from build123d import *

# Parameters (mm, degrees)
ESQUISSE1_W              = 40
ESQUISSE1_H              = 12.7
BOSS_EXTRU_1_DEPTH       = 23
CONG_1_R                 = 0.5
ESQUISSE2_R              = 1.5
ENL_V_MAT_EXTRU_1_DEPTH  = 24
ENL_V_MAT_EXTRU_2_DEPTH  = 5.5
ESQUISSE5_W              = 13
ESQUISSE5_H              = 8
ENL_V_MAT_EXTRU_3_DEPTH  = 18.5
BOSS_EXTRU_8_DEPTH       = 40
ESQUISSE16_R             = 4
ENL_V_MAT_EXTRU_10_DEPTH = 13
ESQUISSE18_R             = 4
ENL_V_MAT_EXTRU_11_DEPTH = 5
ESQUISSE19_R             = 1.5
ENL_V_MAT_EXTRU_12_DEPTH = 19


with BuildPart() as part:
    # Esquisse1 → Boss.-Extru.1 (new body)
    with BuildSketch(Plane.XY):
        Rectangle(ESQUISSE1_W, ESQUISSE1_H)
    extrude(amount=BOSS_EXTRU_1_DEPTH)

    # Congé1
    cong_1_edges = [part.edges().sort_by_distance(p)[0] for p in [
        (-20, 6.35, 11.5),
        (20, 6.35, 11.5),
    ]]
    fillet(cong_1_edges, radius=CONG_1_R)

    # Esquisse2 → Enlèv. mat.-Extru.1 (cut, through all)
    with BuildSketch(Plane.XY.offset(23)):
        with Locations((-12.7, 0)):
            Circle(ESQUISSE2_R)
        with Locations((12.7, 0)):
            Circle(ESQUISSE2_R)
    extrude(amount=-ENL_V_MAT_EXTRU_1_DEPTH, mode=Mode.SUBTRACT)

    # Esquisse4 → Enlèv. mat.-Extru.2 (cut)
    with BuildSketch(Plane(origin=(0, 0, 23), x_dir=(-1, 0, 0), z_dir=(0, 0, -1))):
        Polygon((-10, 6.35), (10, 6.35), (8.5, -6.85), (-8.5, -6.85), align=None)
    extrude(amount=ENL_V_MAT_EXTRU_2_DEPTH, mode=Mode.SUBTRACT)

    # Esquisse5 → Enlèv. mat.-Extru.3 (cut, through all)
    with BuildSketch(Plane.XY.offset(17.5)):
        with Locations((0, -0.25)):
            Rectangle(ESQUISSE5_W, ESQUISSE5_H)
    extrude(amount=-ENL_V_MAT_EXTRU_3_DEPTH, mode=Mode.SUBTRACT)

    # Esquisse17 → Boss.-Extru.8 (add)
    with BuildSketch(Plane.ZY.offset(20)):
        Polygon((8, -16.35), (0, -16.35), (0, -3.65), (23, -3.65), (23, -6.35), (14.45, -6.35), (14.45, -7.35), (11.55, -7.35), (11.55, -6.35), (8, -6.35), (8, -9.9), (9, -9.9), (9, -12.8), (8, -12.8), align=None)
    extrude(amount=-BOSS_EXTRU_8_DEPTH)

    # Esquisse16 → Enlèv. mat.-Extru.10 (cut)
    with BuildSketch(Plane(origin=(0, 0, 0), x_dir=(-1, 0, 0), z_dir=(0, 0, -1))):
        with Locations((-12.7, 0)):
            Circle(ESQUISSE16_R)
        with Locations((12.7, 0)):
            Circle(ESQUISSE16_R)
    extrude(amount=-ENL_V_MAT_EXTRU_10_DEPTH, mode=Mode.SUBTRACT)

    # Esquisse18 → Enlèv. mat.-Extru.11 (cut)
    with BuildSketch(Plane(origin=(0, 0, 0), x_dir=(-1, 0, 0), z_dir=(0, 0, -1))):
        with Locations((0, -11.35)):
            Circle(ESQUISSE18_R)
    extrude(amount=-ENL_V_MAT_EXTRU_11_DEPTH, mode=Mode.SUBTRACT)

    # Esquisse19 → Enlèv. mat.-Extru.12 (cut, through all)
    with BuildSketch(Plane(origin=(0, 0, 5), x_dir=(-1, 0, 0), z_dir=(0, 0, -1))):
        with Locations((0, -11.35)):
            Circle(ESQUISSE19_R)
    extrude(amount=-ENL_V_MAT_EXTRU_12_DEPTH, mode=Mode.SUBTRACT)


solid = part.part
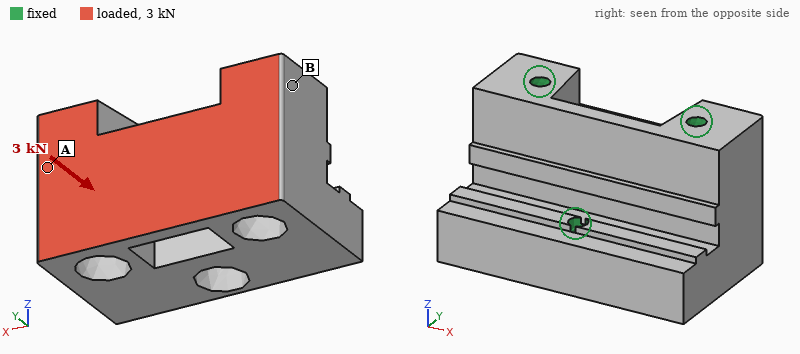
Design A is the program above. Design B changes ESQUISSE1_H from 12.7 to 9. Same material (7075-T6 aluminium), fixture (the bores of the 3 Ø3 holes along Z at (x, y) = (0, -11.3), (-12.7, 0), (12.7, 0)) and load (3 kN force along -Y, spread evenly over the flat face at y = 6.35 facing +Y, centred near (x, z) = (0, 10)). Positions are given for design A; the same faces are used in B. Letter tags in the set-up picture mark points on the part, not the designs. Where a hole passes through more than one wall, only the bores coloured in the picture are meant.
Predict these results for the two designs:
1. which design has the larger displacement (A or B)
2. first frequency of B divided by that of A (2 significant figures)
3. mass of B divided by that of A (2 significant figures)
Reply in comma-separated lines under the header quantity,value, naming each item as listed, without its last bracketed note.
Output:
quantity,value
which design has the larger displacement,B
first frequency of B divided by that of A,0.92
mass of B divided by that of A,0.86
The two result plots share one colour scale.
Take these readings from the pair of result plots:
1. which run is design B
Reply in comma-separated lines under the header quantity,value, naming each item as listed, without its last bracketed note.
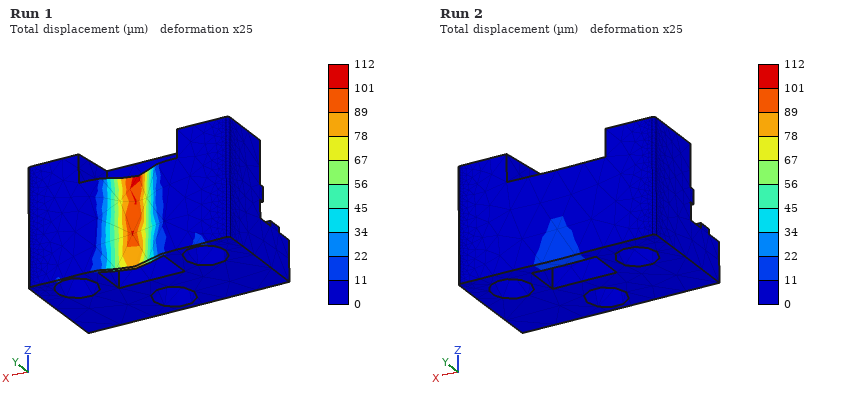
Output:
quantity,value
which run is design B,Run 1
